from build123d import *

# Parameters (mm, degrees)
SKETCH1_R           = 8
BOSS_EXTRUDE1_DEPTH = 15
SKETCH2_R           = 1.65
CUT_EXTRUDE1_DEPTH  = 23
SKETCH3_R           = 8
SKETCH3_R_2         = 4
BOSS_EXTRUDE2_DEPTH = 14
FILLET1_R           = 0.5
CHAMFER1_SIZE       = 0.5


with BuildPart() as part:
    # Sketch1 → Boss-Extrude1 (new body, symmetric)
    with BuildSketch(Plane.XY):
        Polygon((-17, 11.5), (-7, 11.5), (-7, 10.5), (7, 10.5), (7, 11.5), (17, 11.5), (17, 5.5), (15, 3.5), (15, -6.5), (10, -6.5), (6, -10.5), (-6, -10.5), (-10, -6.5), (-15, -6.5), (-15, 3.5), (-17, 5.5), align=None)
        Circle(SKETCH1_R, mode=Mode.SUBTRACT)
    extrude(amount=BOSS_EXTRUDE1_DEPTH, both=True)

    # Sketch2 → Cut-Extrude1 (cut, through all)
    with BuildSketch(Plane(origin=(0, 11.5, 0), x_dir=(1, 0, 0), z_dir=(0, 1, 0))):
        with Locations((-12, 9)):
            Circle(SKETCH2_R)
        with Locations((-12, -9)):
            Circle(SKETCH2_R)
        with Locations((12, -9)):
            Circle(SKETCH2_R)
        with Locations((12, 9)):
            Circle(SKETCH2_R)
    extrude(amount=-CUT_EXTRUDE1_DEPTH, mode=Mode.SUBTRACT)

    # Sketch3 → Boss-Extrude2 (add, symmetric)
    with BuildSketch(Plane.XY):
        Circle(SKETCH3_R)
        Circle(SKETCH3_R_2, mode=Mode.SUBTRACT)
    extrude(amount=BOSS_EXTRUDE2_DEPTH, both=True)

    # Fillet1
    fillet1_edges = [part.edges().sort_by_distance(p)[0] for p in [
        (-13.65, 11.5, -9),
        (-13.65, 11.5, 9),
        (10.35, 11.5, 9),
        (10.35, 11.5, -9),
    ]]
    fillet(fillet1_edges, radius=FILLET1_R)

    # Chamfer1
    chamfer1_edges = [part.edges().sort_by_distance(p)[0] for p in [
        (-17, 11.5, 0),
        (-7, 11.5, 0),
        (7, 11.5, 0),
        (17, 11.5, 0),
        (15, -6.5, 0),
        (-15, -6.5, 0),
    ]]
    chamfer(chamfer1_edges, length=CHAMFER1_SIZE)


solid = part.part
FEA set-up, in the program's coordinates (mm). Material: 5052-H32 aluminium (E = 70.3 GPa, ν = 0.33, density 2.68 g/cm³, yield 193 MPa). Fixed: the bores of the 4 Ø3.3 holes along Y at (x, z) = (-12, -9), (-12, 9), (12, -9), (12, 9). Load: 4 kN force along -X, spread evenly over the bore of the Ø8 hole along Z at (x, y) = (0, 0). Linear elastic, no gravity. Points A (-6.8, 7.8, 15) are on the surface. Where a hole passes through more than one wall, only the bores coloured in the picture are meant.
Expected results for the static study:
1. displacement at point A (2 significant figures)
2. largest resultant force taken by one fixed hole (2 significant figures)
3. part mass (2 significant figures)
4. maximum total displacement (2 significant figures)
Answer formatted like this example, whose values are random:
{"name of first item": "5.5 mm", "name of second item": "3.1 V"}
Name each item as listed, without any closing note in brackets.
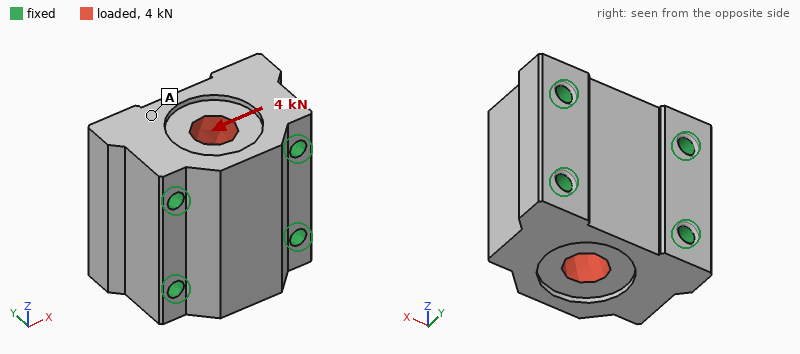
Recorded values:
{"displacement at point A": "0.29 µm", "largest resultant force taken by one fixed hole": "1.0 kN", "part mass": "43 g", "maximum total displacement": "1.2 µm"}
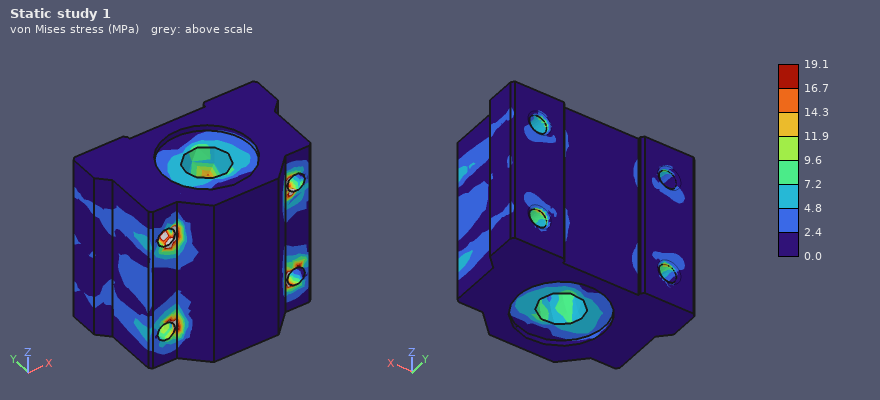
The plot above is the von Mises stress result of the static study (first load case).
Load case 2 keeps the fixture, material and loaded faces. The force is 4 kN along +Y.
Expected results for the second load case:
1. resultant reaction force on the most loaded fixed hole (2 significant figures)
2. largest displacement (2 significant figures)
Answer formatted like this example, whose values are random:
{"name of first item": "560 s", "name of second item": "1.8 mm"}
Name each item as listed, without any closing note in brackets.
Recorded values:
{"resultant reaction force on the most loaded fixed hole": "1.0 kN", "largest displacement": "2.2 µm"}
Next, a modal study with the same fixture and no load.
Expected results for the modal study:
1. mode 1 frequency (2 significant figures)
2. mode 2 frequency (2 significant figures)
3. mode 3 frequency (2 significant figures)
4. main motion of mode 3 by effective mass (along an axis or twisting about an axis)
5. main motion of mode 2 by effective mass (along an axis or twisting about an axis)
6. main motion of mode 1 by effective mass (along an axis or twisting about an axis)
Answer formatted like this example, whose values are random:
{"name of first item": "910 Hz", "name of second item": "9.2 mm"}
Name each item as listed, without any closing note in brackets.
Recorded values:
{"mode 1 frequency": "52 kHz", "mode 2 frequency": "55 kHz", "mode 3 frequency": "63 kHz", "main motion of mode 3 by effective mass": "along Z", "main motion of mode 2 by effective mass": "along Y", "main motion of mode 1 by effective mass": "along Z"}
